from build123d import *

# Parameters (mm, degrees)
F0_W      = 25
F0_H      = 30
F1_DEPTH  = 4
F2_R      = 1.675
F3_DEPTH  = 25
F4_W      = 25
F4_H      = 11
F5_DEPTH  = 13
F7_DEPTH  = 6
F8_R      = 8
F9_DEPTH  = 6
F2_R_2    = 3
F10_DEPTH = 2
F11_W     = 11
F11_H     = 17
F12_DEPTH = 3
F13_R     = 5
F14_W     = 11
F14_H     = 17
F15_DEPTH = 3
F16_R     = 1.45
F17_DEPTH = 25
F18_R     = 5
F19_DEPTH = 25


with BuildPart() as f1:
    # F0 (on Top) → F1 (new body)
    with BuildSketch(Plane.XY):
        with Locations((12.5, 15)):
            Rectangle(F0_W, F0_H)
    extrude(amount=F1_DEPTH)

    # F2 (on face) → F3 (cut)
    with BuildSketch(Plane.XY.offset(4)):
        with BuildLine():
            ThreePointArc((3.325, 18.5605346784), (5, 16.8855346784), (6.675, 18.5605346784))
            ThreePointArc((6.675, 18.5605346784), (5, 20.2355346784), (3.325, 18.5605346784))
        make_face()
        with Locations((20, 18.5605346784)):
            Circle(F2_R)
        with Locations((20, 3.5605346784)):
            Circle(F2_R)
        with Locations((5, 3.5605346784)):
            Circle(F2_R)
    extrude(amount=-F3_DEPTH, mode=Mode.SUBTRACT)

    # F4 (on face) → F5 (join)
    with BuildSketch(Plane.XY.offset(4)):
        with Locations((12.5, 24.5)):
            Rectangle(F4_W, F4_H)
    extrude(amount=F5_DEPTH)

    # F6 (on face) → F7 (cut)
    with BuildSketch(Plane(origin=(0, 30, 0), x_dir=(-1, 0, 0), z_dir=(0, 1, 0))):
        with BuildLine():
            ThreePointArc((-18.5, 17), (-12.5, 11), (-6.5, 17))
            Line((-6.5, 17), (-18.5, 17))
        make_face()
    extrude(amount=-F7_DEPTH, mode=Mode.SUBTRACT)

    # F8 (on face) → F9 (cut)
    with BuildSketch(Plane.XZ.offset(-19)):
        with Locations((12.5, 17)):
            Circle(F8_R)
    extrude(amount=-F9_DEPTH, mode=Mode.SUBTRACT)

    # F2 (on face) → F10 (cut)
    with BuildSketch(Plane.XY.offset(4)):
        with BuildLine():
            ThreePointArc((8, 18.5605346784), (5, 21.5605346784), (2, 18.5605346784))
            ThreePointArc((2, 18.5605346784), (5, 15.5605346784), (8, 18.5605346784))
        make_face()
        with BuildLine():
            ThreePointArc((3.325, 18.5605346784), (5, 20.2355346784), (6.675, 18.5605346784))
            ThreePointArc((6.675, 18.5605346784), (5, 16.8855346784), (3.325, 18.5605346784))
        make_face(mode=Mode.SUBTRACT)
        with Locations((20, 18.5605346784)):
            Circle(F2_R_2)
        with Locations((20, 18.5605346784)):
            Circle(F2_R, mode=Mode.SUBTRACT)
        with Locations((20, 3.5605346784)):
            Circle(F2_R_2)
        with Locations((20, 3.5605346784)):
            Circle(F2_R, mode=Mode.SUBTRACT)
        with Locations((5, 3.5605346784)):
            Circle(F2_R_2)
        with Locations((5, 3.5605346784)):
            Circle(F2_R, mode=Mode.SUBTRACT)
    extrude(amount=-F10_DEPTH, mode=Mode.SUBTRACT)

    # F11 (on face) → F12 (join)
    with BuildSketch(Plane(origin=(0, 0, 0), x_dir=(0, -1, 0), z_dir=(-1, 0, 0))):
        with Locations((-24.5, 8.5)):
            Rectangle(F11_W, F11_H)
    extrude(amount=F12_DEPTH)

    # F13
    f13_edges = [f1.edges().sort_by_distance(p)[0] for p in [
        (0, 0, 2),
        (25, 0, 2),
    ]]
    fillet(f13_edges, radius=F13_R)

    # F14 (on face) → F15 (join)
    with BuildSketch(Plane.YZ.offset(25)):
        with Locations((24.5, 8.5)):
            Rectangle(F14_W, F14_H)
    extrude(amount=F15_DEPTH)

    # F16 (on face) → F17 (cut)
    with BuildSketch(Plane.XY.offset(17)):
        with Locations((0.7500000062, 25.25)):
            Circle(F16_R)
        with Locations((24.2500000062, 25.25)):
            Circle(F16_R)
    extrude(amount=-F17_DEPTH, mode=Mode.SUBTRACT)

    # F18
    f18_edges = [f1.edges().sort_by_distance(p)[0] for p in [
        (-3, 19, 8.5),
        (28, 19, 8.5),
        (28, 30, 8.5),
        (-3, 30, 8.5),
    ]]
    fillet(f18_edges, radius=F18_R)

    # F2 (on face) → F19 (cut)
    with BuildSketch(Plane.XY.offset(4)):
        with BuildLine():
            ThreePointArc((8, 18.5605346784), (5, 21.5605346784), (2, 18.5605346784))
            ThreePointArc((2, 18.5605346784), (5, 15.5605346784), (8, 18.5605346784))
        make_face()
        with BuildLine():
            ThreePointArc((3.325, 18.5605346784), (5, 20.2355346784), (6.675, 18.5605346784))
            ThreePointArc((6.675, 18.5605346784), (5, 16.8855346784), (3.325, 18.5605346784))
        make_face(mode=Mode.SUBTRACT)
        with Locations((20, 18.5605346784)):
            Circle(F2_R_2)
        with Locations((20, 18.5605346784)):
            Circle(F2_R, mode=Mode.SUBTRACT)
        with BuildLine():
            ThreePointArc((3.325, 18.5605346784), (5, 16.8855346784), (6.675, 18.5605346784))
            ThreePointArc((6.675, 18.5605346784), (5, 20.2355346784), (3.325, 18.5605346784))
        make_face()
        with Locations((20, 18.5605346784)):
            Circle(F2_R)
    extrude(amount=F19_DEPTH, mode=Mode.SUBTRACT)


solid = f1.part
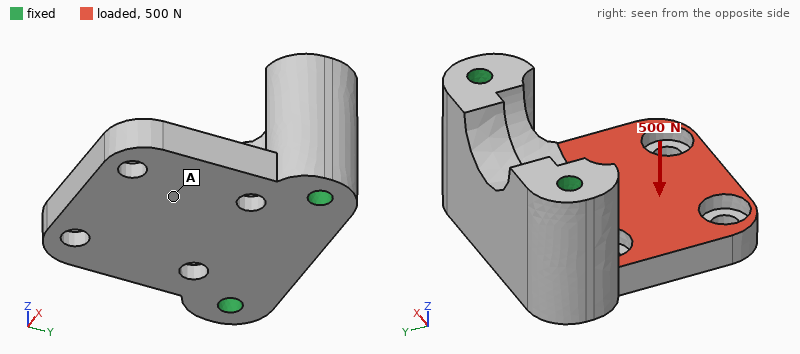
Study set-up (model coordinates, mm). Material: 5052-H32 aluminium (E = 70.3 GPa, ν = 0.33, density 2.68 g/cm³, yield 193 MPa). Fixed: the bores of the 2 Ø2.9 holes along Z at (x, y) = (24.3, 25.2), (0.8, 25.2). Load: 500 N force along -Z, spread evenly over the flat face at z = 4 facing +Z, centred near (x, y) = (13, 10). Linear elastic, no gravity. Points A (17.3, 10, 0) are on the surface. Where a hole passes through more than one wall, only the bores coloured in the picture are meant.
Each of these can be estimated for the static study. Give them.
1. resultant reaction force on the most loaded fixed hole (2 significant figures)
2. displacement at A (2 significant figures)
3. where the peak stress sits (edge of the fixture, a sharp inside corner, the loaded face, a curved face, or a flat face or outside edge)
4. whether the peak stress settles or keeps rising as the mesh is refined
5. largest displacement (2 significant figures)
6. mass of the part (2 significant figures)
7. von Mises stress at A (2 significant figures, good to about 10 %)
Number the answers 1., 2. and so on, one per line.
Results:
1. 250 N
2. 43 µm
3. a sharp inside corner
4. keeps rising
5. 96 µm
6. 15 g
7. 16 MPa
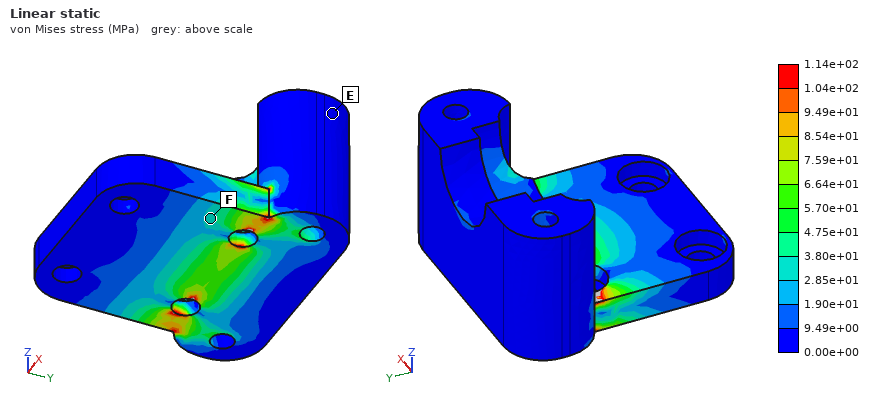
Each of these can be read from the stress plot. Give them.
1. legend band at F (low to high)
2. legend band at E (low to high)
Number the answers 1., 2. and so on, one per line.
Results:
1. 2.85e+01 to 3.80e+01 MPa
2. 0.00e+00 to 9.49e+00 MPa
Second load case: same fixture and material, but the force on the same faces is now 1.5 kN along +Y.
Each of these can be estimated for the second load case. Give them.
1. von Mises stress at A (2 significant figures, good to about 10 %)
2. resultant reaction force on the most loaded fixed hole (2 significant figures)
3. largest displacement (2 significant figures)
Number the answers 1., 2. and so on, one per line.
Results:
1. 15 MPa
2. 760 N
3. 67 µm
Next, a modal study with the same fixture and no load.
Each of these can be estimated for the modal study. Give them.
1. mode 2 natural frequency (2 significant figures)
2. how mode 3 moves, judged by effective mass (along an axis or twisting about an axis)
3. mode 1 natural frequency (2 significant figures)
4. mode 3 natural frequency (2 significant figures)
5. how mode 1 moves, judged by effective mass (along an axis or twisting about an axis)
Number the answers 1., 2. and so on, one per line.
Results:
1. 15 kHz
2. along X
3. 7000 Hz
4. 24 kHz
5. along Z
